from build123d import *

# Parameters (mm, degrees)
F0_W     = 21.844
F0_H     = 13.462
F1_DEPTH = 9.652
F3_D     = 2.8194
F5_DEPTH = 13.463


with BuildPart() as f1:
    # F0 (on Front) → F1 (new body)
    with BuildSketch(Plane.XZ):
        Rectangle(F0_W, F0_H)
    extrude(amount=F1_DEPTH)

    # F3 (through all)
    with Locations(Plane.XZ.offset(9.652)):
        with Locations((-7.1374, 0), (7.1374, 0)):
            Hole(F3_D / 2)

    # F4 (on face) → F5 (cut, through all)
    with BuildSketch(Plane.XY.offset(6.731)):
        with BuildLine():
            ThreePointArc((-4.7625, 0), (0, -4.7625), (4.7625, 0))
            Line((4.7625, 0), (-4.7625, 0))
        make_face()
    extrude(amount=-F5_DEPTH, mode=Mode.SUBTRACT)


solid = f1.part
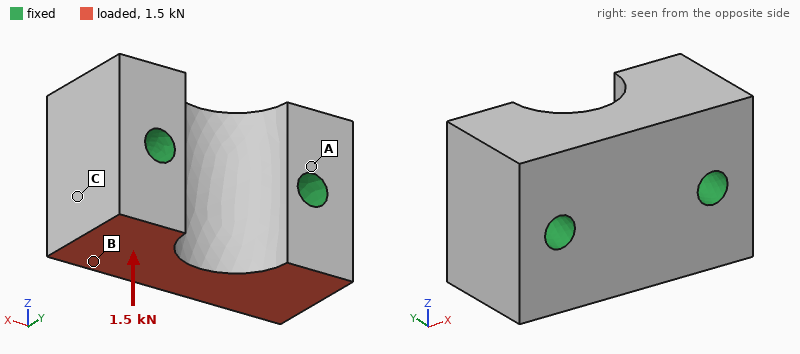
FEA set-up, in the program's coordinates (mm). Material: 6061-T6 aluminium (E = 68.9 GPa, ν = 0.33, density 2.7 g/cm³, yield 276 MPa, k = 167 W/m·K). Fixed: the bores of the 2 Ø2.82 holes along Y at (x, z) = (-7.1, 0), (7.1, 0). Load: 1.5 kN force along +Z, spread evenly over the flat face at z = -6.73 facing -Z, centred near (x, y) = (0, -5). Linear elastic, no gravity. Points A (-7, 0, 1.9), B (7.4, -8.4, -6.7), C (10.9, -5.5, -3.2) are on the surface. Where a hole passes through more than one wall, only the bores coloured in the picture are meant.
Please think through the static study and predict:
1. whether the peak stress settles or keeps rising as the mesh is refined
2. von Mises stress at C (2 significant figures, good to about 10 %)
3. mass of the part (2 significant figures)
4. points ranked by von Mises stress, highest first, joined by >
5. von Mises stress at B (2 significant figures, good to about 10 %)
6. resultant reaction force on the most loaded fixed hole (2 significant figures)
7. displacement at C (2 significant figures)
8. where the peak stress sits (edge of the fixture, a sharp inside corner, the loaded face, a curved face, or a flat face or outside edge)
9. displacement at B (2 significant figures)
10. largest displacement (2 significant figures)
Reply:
keeps rising
5.9 MPa
6.0 g
B > C > A
9.9 MPa
750 N
0.54 µm
edge of the fixture
0.93 µm
1.5 µm
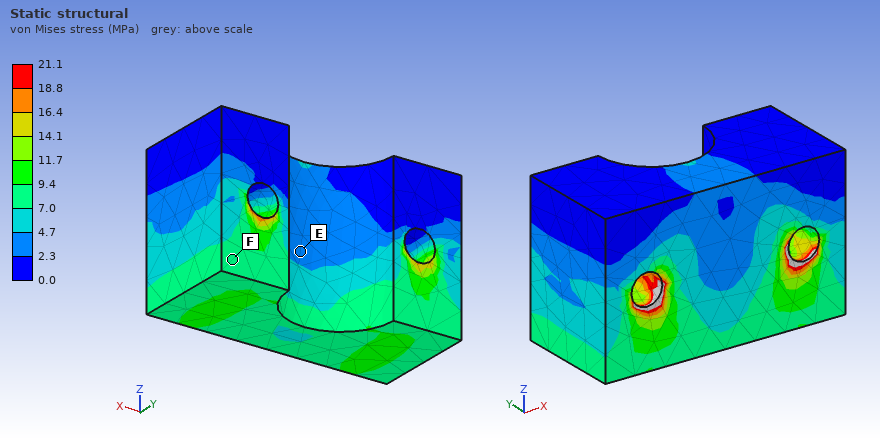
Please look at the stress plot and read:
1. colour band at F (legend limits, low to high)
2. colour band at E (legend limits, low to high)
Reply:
7.0 to 9.4 MPa
2.3 to 4.7 MPa
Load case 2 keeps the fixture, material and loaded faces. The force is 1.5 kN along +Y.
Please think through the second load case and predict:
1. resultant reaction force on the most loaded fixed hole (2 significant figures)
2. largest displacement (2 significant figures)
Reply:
750 N
6.5 µm
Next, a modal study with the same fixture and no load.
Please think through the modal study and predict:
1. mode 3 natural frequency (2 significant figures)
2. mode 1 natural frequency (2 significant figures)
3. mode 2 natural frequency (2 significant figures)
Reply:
85 kHz
76 kHz
84 kHz
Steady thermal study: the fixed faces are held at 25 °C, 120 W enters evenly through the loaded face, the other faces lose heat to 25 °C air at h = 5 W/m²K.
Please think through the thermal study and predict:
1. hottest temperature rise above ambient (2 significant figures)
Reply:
30 K
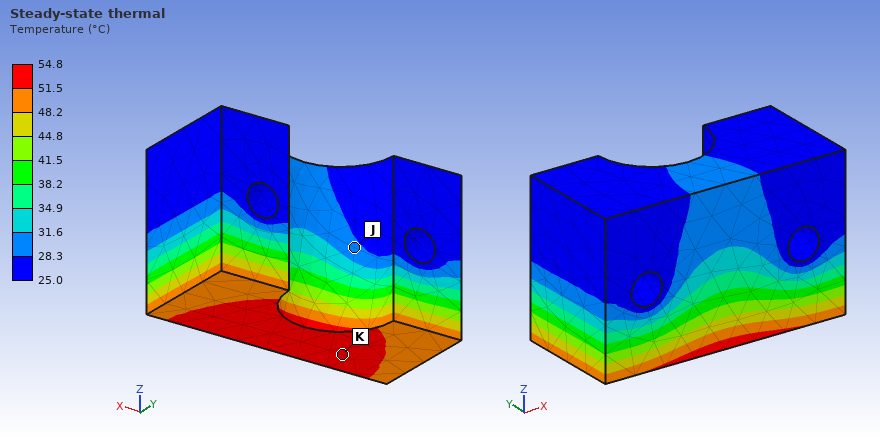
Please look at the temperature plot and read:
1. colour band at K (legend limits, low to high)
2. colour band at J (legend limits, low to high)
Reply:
51.5 to 54.8 °C
28.3 to 31.6 °C
